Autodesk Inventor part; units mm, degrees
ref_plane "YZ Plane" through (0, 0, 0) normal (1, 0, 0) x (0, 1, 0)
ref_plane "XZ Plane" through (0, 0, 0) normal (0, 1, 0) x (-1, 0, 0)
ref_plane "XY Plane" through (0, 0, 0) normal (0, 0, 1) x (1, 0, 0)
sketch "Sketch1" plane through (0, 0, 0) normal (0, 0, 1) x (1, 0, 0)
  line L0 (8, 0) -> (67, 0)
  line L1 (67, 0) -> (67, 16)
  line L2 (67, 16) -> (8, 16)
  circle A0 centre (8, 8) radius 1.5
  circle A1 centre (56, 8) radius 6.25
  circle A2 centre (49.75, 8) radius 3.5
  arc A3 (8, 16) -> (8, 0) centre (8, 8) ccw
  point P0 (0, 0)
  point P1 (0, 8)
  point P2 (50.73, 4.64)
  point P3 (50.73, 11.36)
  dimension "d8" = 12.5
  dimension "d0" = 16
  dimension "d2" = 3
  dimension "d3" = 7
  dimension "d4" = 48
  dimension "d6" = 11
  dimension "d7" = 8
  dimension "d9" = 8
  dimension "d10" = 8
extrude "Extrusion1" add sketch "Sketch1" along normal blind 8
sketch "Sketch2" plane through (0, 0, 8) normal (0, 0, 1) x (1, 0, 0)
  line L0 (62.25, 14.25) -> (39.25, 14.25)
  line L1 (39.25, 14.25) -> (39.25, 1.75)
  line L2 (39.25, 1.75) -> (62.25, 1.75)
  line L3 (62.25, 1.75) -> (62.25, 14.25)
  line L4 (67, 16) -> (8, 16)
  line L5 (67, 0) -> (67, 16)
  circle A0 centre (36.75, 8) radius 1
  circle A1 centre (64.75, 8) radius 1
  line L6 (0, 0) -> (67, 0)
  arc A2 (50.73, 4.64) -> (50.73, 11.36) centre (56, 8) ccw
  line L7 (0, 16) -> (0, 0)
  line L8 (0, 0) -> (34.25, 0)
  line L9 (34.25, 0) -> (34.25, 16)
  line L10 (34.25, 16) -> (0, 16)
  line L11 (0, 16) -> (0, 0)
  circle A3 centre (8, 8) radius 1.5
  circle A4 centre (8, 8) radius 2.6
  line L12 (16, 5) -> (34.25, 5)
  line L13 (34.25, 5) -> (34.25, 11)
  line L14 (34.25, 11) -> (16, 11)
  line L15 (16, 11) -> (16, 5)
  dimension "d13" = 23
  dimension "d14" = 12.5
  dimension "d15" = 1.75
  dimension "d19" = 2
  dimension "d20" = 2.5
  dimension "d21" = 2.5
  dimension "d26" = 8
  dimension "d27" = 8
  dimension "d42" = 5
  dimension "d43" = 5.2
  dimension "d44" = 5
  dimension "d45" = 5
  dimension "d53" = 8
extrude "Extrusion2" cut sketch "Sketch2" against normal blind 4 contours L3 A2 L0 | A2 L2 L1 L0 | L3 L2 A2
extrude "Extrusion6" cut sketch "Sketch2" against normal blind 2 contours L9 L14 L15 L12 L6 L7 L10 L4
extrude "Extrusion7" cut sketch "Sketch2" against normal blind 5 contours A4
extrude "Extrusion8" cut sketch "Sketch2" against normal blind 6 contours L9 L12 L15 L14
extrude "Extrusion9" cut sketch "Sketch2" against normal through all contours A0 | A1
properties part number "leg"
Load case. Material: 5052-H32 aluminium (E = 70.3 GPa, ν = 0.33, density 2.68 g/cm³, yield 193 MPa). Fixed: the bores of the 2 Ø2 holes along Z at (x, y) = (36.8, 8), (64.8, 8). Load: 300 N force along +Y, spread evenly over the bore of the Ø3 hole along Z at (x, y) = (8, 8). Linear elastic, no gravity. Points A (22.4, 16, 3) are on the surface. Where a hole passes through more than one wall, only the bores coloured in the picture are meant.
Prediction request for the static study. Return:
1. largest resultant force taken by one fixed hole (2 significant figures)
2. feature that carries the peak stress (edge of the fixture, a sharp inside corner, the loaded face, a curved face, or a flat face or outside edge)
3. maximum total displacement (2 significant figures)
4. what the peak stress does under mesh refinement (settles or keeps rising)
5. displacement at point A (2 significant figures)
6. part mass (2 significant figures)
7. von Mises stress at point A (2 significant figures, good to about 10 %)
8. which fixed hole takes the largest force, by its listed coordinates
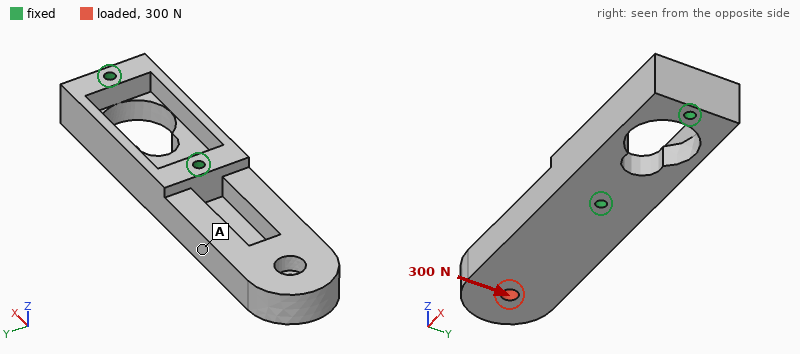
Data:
440 N
edge of the fixture
85 µm
keeps rising
35 µm
13 g
17 MPa
(36.8, 8)
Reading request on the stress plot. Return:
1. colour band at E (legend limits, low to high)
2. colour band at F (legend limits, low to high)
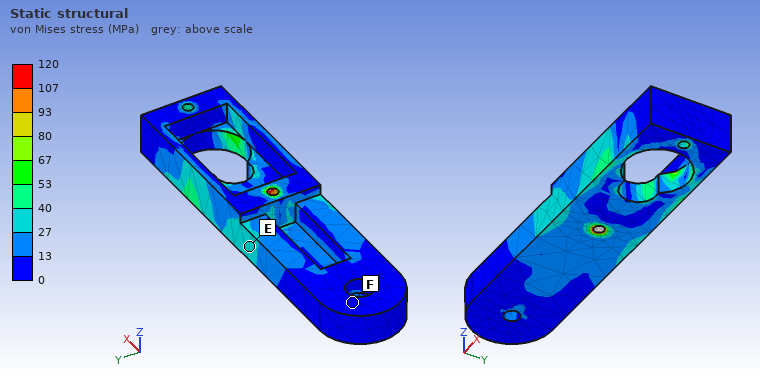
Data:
27 to 40 MPa
0 to 13 MPa
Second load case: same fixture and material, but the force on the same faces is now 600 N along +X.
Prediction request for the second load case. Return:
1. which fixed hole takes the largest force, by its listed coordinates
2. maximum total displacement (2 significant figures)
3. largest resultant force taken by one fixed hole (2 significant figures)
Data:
(36.8, 8)
31 µm
560 N
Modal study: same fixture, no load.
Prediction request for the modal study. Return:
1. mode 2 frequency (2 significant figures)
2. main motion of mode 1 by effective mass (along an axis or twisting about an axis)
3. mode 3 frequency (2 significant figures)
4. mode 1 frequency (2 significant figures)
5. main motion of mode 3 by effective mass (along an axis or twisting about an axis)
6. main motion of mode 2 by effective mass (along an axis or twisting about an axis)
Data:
5200 Hz
along Z
11 kHz
3400 Hz
twisting about X
along Y
